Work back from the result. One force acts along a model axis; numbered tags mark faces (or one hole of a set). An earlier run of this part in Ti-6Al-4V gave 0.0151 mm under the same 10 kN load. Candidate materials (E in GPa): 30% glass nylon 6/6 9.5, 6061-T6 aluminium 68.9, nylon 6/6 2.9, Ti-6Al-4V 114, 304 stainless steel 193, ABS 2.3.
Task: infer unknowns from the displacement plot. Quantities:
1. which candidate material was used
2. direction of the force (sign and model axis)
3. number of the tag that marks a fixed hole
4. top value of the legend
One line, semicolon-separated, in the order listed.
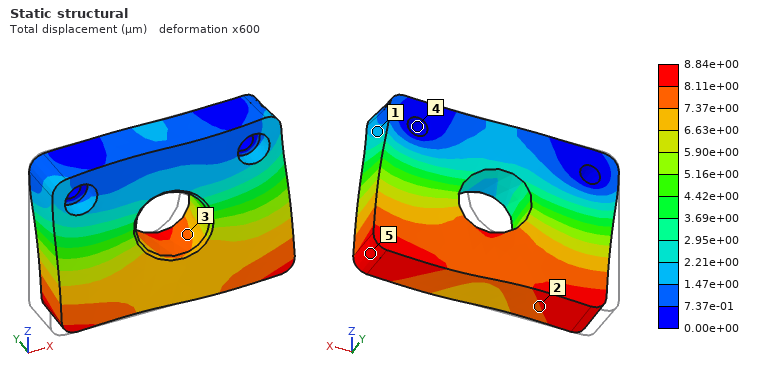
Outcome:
304 stainless steel; +X; 4; 8.84e+00 µm
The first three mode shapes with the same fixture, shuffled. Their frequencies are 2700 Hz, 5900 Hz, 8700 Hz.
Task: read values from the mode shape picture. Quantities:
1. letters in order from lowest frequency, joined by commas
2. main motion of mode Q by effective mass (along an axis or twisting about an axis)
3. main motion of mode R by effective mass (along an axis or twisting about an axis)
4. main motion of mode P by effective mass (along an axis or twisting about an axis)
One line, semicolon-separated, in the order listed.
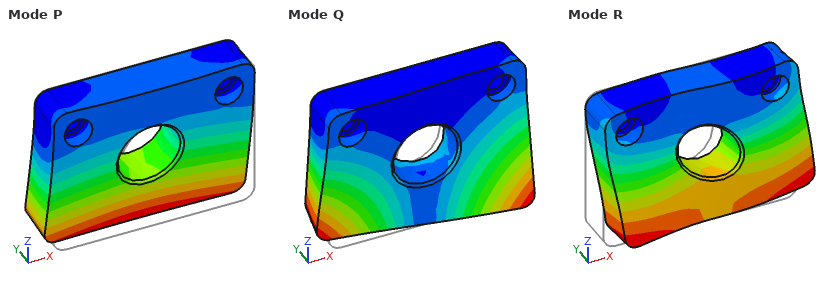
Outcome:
P, Q, R; twisting about Z; along X; along Y
